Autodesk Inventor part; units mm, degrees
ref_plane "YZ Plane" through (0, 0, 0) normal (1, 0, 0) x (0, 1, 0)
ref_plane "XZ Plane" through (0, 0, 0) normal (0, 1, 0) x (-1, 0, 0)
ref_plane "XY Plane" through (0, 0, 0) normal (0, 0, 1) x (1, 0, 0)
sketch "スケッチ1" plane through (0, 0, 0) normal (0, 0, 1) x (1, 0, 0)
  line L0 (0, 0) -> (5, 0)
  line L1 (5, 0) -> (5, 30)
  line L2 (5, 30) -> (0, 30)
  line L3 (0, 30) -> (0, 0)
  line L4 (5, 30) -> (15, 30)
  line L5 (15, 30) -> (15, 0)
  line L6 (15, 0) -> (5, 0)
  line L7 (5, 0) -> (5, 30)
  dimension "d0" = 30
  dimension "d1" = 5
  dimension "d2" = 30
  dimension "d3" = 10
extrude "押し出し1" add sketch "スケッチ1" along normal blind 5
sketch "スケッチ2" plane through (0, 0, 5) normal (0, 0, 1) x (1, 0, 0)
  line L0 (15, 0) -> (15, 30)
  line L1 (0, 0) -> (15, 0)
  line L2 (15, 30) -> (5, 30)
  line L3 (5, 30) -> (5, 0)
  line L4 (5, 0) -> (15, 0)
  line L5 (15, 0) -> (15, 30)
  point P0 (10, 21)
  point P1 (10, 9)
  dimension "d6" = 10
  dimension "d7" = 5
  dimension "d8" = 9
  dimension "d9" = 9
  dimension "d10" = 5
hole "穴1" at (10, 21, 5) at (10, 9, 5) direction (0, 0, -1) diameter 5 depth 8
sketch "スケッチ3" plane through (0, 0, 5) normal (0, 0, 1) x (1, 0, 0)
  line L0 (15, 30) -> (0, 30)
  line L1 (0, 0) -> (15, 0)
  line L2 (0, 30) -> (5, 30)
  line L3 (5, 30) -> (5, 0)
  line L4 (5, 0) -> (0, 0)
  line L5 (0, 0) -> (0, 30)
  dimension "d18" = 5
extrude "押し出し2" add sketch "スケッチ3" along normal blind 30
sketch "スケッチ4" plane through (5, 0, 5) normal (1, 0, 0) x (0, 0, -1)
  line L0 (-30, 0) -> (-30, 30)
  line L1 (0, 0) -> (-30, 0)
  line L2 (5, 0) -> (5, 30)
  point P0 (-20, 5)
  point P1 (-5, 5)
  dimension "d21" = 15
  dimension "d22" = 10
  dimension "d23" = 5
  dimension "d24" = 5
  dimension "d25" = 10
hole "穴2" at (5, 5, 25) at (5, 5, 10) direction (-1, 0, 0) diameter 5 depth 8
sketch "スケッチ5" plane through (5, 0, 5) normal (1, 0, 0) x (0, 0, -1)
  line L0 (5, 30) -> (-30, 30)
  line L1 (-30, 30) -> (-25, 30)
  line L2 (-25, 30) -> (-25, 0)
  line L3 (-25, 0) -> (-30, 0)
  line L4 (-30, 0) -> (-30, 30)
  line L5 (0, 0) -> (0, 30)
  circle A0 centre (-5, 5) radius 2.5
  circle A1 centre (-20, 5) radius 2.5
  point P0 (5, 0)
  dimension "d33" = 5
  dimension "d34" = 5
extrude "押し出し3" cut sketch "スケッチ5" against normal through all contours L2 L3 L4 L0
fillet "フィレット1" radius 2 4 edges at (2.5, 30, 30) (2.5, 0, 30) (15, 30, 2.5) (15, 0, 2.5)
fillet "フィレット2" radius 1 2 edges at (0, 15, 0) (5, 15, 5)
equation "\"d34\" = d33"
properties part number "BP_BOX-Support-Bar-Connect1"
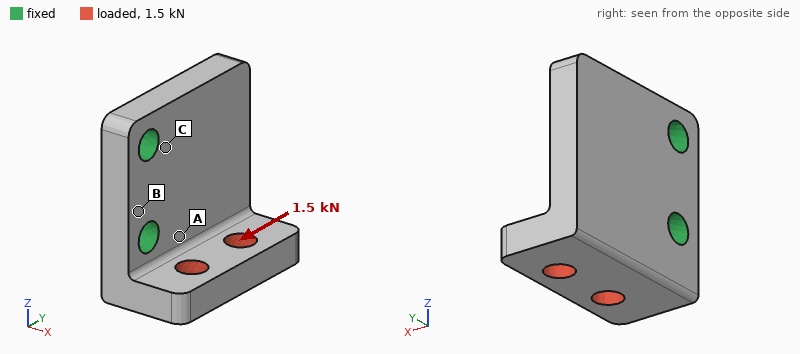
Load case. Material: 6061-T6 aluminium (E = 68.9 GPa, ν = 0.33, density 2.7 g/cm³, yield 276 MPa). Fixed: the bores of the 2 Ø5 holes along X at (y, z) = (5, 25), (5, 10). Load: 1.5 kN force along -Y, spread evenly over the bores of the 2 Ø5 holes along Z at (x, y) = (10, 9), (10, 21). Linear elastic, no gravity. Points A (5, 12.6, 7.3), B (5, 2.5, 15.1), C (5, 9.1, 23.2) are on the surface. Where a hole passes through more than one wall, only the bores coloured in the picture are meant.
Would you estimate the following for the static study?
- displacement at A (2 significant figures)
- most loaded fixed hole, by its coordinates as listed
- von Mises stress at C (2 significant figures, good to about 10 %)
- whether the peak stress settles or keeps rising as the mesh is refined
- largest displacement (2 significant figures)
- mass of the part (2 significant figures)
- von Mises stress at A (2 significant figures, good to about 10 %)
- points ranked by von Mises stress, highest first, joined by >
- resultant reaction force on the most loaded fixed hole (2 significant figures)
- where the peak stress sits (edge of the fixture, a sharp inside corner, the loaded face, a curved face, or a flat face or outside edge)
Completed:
18 µm
(5, 10)
33 MPa
keeps rising
98 µm
15 g
59 MPa
A > C > B
1.9 kN
edge of the fixture
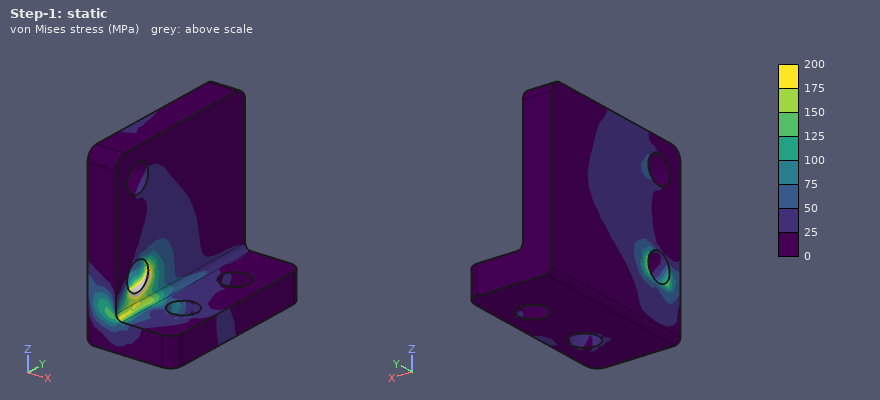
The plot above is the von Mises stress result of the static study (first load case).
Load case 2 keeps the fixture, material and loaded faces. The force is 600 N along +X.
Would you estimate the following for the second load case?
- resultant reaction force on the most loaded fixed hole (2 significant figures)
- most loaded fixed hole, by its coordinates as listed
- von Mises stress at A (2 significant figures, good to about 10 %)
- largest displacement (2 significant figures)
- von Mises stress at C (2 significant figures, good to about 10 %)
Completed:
680 N
(5, 10)
23 MPa
57 µm
19 MPa
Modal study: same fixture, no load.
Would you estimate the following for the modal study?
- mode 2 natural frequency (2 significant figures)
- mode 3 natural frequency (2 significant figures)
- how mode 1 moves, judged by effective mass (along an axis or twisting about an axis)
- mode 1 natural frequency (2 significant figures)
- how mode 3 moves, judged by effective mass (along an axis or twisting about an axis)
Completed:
10 kHz
15 kHz
along X
6500 Hz
along Z
